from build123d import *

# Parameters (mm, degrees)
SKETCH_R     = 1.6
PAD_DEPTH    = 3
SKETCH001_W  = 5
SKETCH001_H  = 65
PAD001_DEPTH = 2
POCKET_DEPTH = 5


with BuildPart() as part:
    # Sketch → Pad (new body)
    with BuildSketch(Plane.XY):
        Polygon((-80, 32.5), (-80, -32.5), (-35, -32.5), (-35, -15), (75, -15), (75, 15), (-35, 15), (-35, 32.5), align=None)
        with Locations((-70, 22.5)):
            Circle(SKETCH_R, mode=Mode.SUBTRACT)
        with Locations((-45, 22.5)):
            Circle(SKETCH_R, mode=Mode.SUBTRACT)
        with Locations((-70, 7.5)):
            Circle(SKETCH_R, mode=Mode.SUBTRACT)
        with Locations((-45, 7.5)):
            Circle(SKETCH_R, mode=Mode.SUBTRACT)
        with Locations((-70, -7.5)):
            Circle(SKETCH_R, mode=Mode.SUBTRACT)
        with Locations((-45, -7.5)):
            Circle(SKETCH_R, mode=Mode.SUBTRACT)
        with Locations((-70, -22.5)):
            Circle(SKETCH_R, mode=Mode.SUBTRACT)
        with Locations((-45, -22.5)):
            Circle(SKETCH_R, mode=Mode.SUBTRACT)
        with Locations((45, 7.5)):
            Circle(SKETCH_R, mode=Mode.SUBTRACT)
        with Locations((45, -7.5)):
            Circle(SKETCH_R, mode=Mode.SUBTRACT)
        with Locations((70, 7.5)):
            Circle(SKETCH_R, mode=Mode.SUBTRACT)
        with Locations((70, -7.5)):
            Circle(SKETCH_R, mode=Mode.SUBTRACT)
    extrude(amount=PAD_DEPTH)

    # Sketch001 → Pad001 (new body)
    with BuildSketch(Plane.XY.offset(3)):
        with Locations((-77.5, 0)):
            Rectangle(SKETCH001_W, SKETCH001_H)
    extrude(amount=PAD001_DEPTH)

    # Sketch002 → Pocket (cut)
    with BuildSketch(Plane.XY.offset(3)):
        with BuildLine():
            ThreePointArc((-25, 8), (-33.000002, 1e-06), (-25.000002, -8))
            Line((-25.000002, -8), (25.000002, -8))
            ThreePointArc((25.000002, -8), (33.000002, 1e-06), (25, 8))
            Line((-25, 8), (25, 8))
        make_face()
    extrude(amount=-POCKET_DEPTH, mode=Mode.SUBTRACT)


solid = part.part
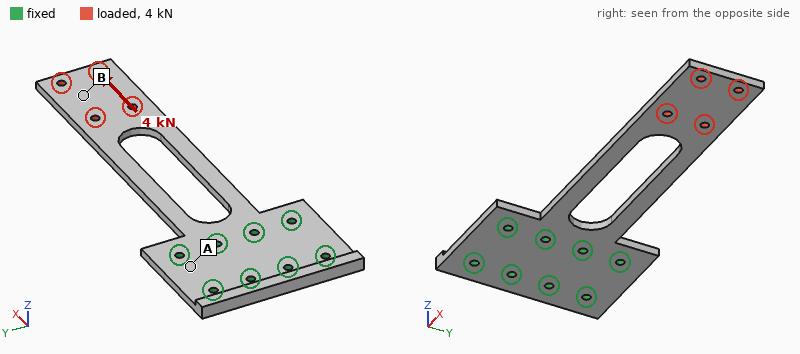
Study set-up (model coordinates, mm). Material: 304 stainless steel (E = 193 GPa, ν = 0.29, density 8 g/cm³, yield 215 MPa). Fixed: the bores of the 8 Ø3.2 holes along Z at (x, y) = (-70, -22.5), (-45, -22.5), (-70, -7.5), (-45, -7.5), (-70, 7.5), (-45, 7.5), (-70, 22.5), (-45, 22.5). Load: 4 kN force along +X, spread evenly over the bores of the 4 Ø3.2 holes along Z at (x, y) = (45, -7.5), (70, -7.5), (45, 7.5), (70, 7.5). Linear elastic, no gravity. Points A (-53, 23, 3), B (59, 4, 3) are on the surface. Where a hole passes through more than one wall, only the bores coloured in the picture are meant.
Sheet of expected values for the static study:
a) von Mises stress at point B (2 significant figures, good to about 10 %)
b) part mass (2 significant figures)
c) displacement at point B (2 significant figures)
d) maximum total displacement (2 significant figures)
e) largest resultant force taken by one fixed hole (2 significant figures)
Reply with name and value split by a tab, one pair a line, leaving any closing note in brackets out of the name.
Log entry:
von Mises stress at point B	20 MPa
part mass	130 g
displacement at point B	43 µm
maximum total displacement	45 µm
largest resultant force taken by one fixed hole	1.3 kN
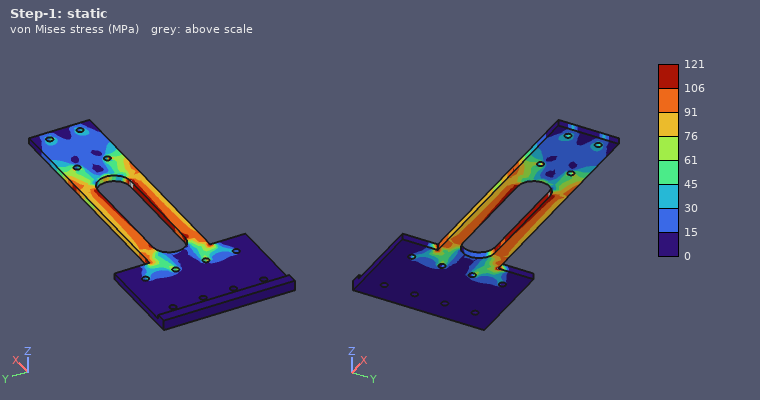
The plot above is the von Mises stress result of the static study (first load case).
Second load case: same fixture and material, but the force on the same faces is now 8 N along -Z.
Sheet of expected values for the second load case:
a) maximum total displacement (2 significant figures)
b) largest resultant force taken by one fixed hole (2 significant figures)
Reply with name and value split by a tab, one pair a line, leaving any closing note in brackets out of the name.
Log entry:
maximum total displacement	0.47 mm
largest resultant force taken by one fixed hole	7.5 N
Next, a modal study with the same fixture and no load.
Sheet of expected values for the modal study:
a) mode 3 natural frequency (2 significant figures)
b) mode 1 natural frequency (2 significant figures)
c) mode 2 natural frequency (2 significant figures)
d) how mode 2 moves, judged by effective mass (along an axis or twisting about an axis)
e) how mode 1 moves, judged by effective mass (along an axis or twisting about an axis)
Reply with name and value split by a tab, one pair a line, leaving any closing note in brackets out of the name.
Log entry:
mode 3 natural frequency	940 Hz
mode 1 natural frequency	140 Hz
mode 2 natural frequency	860 Hz
how mode 2 moves, judged by effective mass	along Y
how mode 1 moves, judged by effective mass	along Z
